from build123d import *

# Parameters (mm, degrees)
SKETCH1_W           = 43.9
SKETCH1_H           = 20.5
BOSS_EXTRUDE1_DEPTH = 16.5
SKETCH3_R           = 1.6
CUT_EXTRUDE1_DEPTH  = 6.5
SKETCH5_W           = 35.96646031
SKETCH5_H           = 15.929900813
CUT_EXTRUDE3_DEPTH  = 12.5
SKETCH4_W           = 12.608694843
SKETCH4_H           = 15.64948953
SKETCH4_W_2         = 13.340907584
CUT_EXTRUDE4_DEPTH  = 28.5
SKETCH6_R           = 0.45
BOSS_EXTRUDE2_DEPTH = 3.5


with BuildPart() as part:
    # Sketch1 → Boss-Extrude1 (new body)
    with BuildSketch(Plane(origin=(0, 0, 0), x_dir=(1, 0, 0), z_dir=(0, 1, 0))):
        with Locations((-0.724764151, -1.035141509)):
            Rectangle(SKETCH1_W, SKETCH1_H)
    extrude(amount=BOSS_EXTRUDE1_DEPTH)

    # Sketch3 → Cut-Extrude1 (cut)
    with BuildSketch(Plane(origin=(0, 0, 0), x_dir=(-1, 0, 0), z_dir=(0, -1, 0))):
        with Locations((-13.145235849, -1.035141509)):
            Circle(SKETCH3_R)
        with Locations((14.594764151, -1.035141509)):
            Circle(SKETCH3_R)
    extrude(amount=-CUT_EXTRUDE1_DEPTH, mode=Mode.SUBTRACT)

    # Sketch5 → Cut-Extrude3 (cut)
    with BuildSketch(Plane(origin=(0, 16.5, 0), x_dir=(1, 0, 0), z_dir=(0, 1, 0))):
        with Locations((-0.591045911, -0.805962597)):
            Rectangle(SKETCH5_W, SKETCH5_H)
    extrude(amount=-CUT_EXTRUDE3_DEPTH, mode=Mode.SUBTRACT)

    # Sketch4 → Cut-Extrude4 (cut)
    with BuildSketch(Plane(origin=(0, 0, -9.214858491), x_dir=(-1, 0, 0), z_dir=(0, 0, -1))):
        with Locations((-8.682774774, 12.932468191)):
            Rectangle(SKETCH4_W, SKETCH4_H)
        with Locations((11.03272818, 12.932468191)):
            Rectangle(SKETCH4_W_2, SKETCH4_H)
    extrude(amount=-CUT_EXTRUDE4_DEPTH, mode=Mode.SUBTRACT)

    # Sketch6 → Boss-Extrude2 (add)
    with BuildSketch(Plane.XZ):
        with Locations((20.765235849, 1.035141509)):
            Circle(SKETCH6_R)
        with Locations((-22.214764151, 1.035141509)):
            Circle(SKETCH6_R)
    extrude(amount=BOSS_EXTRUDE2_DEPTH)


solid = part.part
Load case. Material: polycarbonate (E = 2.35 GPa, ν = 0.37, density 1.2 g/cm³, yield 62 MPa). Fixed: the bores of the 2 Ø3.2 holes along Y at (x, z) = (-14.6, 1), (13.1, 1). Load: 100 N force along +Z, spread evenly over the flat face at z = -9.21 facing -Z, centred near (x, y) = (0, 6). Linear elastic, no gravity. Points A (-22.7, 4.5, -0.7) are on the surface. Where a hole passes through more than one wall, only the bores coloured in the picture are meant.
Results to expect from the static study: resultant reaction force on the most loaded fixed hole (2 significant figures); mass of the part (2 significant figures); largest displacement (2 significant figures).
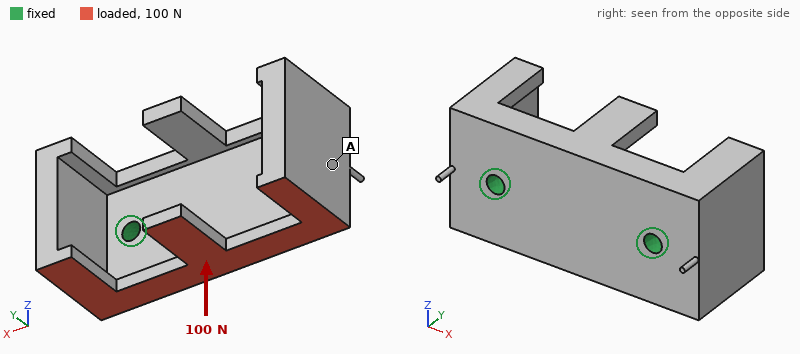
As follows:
52 N
7.5 g
0.60 mm
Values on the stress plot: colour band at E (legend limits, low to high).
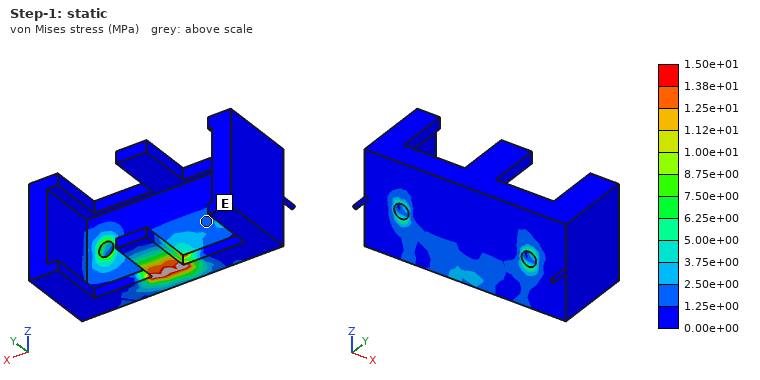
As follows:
1.25e+00 to 2.50e+00 MPa
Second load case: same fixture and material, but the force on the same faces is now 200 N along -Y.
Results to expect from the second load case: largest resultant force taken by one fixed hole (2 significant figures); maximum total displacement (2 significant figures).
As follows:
100 N
0.58 mm
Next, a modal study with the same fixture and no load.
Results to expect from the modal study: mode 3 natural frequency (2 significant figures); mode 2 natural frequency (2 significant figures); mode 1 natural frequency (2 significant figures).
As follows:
2800 Hz
2600 Hz
2400 Hz
